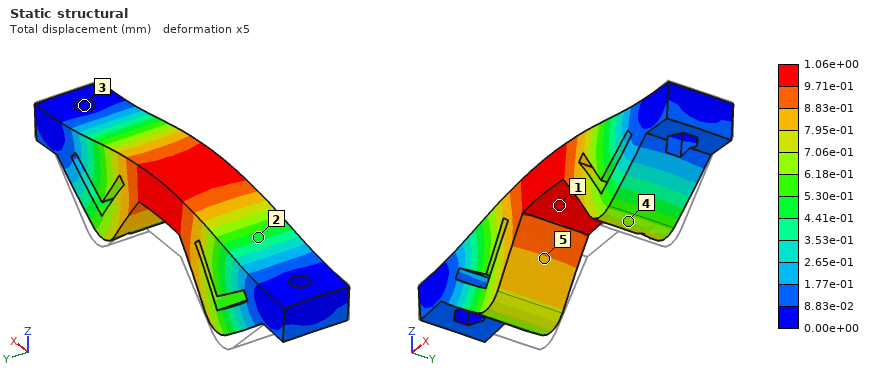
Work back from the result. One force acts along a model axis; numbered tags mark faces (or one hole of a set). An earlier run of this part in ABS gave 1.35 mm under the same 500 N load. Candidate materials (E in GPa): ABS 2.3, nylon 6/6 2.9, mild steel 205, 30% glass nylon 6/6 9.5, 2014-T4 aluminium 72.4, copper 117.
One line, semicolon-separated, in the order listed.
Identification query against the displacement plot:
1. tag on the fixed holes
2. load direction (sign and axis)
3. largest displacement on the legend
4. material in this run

3; +Z; 1.06e+00 mm; nylon 6/6
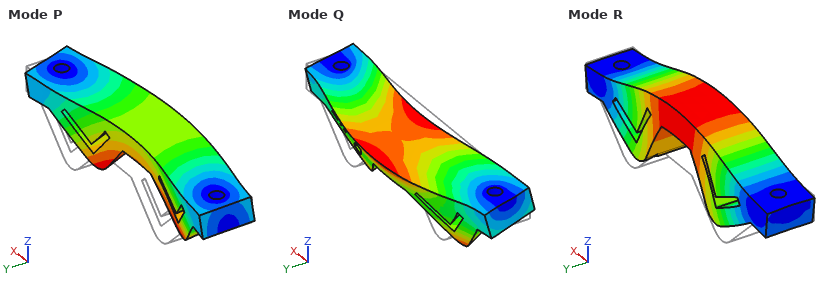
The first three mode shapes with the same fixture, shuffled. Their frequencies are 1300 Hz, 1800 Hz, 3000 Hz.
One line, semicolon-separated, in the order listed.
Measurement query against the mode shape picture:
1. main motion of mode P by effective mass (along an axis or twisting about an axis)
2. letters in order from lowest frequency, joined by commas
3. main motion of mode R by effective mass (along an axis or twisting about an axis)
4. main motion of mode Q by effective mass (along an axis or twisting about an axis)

along Y; R, P, Q; along Z; twisting about X
